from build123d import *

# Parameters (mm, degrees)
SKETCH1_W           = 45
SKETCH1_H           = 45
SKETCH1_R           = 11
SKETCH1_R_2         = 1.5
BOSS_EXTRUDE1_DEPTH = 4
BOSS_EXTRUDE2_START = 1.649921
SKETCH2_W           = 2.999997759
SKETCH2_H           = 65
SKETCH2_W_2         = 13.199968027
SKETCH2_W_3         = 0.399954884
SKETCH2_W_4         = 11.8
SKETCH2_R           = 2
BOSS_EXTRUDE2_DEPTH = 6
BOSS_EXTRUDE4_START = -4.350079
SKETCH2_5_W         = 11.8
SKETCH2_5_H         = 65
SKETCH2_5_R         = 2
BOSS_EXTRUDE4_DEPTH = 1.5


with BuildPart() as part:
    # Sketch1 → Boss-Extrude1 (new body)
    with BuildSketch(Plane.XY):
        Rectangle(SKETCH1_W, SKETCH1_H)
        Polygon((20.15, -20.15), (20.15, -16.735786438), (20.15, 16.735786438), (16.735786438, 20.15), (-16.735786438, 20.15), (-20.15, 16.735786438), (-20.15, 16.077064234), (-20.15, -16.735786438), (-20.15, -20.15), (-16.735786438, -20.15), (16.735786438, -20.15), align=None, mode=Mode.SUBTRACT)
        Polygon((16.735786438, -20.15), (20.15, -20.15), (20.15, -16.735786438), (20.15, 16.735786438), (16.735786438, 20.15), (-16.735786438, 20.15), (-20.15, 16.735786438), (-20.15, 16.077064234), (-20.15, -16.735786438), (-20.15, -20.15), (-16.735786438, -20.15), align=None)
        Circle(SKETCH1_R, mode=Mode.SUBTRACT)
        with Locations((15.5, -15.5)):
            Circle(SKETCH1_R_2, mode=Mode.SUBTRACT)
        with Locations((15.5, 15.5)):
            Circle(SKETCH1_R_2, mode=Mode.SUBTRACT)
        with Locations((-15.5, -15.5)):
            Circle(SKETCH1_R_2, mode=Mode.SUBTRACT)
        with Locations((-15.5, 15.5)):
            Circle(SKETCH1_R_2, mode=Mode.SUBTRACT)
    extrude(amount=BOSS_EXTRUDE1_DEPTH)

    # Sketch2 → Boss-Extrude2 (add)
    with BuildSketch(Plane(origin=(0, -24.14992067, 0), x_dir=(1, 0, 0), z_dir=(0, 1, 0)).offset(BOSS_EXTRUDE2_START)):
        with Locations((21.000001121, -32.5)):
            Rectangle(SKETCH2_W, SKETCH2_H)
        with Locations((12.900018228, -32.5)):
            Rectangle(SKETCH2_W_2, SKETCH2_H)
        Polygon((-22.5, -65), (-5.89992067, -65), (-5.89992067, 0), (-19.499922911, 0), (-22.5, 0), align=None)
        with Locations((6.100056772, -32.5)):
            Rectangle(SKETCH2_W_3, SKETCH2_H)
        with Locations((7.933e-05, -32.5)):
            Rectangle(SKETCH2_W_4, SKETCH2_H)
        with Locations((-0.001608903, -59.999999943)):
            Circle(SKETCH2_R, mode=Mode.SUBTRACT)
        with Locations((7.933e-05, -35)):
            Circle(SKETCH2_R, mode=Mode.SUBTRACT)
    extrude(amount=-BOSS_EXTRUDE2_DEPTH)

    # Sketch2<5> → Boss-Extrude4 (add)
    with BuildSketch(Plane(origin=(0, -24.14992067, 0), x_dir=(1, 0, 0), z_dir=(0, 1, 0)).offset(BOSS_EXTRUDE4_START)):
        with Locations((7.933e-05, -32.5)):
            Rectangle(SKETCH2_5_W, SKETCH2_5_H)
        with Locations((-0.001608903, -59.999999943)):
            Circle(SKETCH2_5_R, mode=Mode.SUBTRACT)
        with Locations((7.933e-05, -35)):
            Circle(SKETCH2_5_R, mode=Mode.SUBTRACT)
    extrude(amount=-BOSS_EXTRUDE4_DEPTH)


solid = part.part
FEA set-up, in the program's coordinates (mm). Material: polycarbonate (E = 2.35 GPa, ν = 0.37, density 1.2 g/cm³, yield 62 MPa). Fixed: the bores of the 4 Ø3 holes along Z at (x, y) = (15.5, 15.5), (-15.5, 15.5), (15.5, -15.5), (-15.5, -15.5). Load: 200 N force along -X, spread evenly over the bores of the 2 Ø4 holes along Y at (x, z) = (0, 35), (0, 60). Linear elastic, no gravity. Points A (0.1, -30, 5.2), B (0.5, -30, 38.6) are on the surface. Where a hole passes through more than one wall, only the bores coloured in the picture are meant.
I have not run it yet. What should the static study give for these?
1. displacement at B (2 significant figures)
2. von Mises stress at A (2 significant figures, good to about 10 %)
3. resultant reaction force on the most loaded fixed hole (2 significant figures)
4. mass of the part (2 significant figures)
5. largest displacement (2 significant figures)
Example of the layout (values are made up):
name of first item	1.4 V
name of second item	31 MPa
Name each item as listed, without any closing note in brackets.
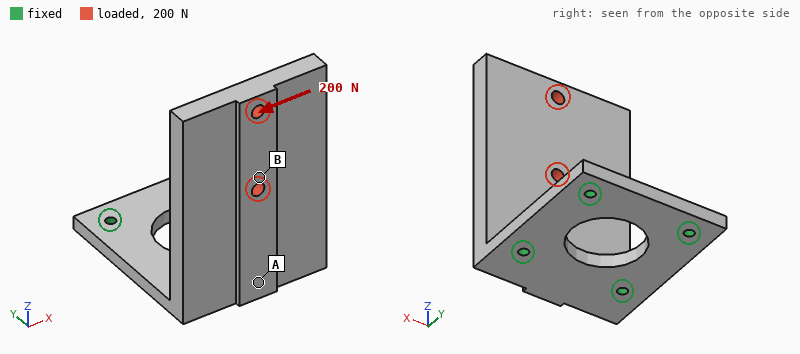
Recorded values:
displacement at B	0.52 mm
von Mises stress at A	6.4 MPa
resultant reaction force on the most loaded fixed hole	310 N
mass of the part	30 g
largest displacement	1.1 mm
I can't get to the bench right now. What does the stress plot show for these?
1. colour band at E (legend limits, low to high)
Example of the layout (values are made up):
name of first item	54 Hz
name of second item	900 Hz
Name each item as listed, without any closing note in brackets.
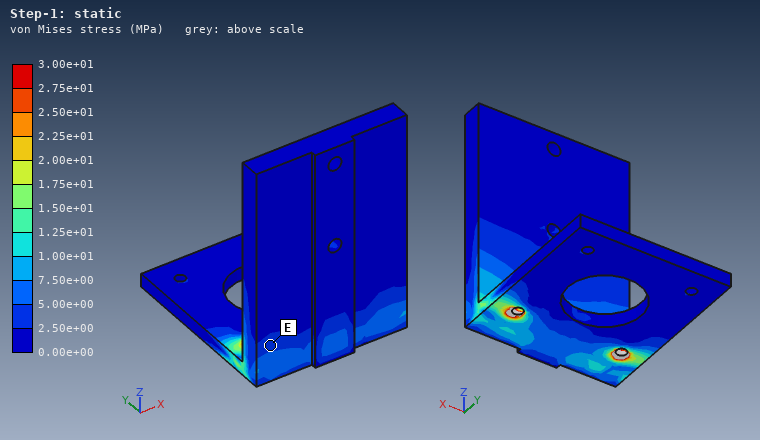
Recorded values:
colour band at E	2.50e+00 to 5.00e+00 MPa
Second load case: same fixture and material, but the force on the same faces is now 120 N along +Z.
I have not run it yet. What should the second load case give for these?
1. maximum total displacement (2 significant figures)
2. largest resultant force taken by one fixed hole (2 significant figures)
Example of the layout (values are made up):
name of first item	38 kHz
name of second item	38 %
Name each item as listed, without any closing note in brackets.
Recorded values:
maximum total displacement	0.99 mm
largest resultant force taken by one fixed hole	64 N
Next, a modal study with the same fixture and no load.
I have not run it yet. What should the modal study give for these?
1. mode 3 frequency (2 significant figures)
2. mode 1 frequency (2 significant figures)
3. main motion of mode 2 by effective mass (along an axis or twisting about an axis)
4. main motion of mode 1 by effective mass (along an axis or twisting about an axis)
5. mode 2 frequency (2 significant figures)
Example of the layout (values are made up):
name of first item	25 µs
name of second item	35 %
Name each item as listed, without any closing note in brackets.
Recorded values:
mode 3 frequency	1100 Hz
mode 1 frequency	190 Hz
main motion of mode 2 by effective mass	along X
main motion of mode 1 by effective mass	along Y
mode 2 frequency	660 Hz
